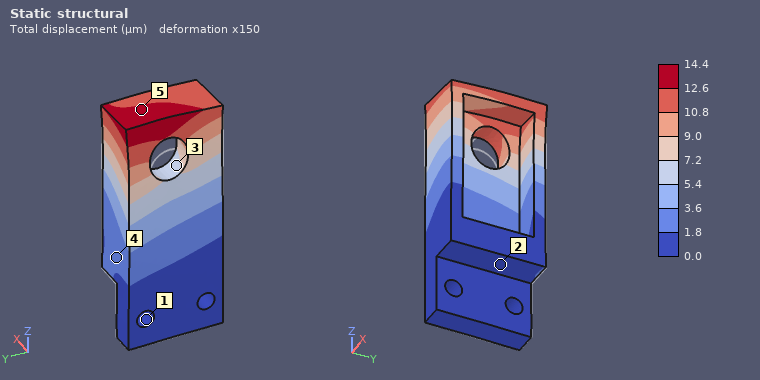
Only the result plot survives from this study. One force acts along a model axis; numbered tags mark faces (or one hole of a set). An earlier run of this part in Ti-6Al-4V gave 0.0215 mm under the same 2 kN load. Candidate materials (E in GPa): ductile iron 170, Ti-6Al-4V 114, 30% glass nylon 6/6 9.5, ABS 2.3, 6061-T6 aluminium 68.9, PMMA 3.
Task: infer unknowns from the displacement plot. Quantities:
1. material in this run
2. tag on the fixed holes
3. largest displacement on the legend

ductile iron
1
14.4 µm
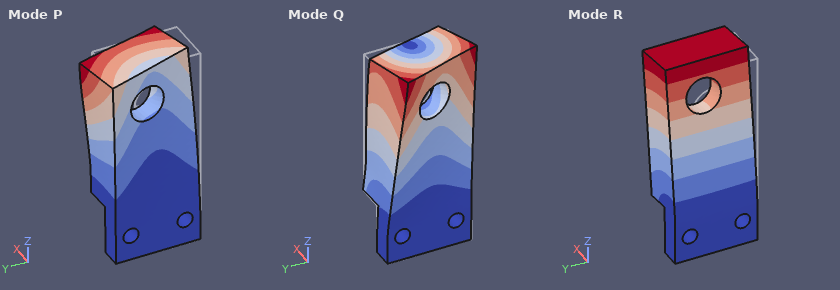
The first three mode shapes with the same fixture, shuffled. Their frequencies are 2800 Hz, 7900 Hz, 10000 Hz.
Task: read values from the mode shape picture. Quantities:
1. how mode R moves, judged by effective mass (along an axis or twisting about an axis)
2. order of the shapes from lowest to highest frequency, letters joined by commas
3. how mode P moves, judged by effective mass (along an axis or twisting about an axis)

along X
R, P, Q
along Y
